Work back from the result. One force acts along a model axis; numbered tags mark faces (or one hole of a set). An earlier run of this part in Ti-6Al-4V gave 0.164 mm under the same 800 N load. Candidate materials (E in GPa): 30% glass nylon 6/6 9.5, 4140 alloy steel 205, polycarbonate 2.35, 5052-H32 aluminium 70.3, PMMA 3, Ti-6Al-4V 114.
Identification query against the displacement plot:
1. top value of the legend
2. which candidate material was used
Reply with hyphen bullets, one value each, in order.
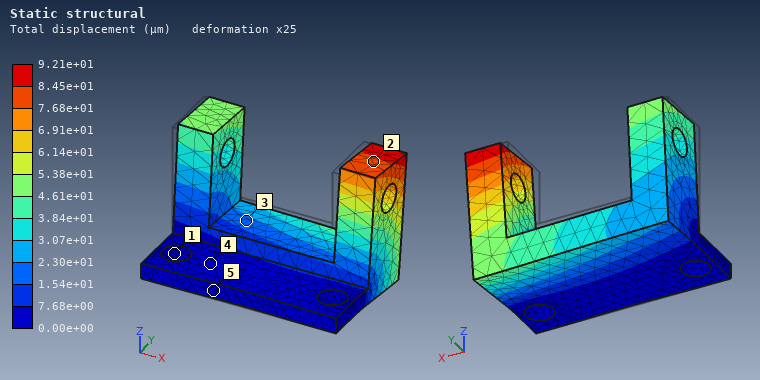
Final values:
- 9.21e+01 µm
- 4140 alloy steel
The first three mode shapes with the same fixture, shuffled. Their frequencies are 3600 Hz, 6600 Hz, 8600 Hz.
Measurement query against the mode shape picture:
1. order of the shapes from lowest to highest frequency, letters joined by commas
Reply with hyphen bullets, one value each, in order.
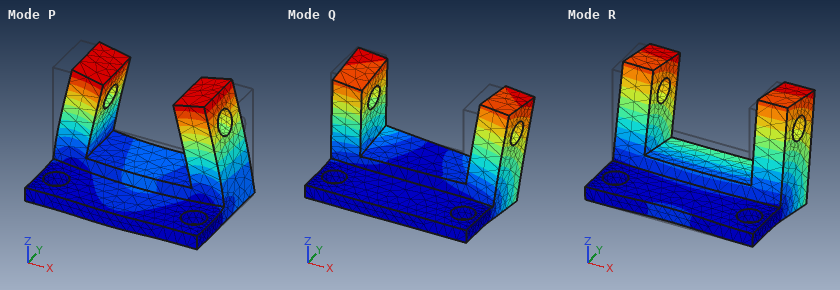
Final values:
- R, Q, P
